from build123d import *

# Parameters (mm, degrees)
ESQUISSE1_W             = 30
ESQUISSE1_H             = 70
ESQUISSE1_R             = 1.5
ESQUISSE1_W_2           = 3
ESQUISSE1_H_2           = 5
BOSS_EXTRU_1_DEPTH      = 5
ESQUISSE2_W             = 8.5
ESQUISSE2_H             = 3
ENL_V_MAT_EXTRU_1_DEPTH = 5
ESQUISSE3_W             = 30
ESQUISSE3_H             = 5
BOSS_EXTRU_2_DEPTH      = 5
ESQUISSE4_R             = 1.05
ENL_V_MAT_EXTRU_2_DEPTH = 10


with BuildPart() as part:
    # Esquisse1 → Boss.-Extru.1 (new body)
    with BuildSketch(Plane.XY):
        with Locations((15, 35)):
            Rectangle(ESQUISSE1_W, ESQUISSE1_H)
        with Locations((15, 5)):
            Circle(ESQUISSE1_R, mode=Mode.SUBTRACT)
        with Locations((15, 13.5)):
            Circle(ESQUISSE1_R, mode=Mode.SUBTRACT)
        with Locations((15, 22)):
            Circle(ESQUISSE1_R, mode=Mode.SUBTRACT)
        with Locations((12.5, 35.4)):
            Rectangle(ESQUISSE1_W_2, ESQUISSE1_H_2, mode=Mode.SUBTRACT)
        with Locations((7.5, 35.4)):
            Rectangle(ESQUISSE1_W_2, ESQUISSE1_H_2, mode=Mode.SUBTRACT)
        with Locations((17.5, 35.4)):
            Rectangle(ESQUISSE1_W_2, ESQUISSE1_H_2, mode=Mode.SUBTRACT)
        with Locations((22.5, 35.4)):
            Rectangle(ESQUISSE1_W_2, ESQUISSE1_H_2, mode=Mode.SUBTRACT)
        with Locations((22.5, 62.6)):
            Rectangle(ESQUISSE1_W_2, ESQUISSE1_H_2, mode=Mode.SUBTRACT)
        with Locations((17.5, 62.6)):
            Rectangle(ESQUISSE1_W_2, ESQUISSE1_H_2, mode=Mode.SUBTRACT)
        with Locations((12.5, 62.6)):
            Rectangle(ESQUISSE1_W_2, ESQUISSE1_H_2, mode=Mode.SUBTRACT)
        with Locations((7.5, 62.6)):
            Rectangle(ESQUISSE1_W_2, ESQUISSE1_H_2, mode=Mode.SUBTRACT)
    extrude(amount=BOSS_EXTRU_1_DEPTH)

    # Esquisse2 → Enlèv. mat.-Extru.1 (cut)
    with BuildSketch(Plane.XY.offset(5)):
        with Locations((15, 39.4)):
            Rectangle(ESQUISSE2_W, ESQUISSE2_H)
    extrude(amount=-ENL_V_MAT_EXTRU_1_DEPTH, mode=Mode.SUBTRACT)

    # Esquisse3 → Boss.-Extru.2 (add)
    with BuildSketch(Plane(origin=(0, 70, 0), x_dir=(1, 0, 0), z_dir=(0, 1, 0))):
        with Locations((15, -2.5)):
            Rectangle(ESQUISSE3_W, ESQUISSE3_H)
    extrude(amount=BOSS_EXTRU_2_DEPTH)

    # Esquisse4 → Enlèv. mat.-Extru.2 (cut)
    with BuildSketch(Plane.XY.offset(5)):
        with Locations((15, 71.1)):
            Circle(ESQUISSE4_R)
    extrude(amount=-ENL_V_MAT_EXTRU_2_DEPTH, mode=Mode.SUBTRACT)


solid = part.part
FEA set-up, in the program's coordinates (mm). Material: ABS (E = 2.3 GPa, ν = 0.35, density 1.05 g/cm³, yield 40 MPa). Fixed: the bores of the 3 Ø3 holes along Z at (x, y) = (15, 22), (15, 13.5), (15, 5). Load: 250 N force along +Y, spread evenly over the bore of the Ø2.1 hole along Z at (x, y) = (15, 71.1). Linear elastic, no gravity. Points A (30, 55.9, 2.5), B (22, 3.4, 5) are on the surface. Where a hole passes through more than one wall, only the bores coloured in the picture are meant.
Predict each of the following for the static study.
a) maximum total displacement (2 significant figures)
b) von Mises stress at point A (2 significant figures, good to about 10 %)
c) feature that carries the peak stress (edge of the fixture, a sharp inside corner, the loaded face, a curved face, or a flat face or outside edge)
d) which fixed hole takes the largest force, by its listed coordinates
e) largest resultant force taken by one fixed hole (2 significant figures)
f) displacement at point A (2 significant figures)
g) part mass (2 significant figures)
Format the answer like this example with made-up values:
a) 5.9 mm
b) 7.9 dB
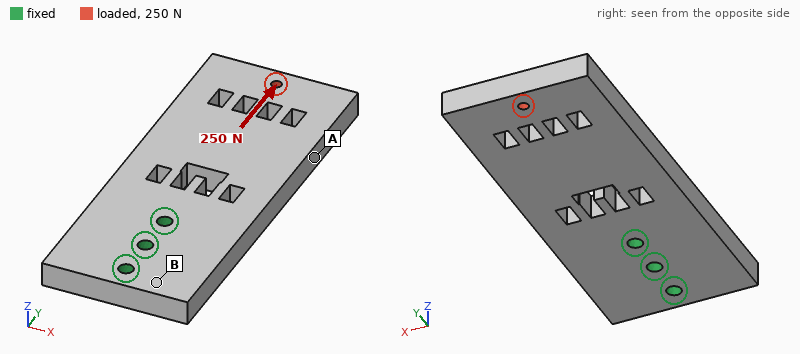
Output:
a) 88 µm
b) 1.8 MPa
c) the loaded face
d) (15, 22)
e) 140 N
f) 42 µm
g) 11 g
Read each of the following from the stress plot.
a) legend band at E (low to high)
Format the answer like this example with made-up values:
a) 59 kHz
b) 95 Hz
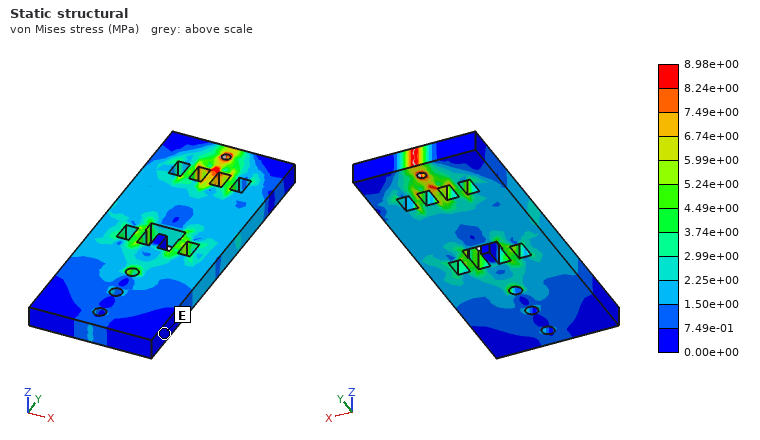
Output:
a) 0.00e+00 to 7.49e-01 MPa
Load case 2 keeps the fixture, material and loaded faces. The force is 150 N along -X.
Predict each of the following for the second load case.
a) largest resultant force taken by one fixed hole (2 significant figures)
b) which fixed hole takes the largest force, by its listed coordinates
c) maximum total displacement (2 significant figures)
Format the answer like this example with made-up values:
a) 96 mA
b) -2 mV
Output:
a) 540 N
b) (15, 22)
c) 0.78 mm
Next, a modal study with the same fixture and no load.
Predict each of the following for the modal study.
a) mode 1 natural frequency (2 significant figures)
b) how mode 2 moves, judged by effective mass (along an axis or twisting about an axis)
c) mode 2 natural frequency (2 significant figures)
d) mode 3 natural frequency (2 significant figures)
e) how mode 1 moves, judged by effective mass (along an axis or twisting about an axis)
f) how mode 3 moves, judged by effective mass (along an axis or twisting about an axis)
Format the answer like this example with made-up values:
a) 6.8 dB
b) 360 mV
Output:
a) 370 Hz
b) twisting about Y
c) 1200 Hz
d) 1300 Hz
e) along Z
f) along X
